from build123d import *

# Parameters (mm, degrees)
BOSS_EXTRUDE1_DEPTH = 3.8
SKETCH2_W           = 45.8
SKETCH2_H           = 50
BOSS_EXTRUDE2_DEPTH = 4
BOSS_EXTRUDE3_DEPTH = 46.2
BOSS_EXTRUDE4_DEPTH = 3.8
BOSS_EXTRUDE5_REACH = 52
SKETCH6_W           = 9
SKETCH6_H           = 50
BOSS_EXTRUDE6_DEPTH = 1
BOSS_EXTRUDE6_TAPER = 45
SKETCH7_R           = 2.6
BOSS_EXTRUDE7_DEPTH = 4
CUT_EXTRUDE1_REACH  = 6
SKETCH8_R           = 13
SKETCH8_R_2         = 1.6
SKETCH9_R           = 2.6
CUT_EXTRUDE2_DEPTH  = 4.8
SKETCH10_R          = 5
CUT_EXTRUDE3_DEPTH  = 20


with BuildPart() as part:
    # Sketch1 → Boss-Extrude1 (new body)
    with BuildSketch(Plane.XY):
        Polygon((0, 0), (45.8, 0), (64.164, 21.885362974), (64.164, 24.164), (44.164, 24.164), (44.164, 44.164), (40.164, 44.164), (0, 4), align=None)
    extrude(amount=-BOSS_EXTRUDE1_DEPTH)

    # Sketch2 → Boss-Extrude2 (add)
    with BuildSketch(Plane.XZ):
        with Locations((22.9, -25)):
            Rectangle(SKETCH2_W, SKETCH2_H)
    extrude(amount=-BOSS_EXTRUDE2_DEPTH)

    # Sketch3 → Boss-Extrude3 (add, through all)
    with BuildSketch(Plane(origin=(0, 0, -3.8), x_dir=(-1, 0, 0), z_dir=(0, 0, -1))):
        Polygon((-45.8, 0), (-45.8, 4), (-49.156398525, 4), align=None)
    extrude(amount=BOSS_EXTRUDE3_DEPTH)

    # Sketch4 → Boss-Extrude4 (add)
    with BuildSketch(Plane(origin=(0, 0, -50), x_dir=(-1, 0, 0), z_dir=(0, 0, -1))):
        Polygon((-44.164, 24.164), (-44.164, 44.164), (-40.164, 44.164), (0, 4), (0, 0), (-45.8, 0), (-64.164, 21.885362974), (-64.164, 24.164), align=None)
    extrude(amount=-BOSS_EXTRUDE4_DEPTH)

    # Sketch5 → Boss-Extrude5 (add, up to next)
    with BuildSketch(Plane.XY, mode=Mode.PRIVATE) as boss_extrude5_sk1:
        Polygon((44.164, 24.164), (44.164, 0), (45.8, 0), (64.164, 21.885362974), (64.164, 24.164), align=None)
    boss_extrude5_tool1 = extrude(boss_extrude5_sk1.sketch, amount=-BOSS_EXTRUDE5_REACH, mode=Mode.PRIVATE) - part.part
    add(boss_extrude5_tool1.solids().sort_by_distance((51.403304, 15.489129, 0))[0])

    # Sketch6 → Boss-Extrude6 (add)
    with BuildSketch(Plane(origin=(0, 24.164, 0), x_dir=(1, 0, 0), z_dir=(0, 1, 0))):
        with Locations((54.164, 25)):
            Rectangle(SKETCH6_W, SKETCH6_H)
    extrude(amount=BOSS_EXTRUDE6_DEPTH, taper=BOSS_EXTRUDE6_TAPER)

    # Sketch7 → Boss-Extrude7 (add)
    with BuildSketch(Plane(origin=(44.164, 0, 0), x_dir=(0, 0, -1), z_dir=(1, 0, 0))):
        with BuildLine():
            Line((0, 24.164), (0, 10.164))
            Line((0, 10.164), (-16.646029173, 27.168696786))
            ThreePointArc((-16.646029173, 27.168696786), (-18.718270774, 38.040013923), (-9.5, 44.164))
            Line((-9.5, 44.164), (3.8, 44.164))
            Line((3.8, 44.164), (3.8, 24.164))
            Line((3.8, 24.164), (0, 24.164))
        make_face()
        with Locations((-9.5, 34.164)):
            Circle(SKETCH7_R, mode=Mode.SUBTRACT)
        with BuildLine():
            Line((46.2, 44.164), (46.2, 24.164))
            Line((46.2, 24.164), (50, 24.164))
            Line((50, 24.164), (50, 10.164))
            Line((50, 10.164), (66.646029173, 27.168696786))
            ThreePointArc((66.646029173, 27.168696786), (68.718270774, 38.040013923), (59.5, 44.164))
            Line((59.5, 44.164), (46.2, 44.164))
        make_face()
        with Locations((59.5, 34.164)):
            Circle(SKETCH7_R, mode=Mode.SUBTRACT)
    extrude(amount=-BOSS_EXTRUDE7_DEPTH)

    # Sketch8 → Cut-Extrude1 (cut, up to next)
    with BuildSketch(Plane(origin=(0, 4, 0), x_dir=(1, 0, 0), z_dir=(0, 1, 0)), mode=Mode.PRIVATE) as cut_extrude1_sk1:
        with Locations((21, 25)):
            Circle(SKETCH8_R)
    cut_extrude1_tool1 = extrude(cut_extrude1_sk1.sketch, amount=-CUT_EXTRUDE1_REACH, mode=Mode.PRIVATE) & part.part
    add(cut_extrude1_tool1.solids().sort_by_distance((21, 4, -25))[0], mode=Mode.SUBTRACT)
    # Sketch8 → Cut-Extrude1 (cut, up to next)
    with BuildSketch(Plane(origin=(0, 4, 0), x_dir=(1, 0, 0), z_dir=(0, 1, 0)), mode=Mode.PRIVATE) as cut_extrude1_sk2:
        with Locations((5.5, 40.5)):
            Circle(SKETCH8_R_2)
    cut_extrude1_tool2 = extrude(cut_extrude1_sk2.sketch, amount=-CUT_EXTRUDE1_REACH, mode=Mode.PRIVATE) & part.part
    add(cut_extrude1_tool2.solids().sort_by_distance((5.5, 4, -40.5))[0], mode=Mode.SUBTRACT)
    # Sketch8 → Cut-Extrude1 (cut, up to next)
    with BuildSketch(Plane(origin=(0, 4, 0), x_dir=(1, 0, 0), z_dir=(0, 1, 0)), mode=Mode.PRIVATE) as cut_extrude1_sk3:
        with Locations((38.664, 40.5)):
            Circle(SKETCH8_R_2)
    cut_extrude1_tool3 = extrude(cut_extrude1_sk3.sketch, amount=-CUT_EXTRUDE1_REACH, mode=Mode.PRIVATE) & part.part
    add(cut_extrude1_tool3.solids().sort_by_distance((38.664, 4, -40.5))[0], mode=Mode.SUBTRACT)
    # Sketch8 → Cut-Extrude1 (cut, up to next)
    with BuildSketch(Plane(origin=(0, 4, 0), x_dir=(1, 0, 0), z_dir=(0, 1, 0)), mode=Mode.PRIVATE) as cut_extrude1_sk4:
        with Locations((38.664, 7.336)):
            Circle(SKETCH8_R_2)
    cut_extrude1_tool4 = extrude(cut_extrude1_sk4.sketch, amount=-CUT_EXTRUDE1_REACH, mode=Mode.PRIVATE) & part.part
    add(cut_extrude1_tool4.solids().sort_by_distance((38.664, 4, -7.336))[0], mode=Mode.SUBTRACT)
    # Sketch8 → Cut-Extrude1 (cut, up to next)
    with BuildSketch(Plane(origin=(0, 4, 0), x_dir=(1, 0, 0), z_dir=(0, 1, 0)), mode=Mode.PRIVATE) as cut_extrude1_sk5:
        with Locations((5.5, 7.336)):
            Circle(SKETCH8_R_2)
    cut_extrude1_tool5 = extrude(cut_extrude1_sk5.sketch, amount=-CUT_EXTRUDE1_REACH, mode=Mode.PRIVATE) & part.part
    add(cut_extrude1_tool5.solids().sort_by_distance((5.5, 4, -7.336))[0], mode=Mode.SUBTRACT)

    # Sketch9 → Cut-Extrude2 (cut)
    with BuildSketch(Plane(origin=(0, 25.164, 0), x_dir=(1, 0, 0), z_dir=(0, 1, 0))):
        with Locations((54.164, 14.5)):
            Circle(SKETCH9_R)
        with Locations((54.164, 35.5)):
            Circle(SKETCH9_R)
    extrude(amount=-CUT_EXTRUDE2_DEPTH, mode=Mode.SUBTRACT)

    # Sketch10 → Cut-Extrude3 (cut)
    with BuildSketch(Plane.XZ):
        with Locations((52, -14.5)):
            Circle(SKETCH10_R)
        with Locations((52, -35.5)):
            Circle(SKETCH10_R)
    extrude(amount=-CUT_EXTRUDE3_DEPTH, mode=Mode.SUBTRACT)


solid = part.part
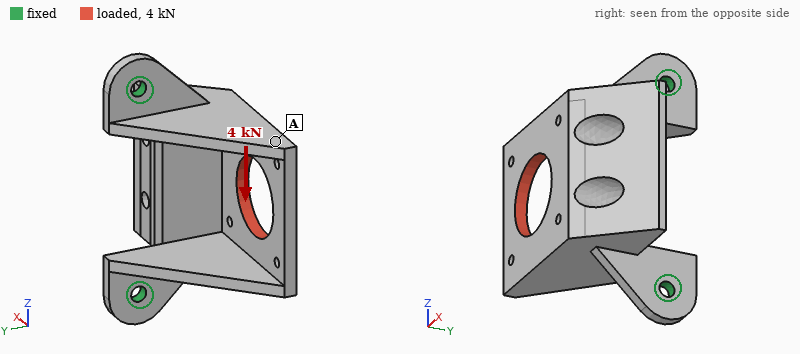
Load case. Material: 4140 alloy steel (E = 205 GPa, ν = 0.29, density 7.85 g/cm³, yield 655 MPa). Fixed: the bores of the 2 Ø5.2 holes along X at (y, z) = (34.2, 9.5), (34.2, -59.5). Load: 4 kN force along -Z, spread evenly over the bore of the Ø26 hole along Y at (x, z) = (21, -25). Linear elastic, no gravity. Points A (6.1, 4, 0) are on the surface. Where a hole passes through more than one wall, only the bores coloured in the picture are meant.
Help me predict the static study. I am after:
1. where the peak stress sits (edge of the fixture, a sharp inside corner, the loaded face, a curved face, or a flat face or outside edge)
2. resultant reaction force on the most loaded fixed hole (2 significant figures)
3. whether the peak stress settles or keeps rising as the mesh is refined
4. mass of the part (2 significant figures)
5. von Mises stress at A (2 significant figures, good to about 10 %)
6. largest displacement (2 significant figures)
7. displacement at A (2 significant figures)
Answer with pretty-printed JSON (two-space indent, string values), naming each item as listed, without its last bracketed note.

{
  "where the peak stress sits": "edge of the fixture",
  "resultant reaction force on the most loaded fixed hole": "2.8 kN",
  "whether the peak stress settles or keeps rising as the mesh is refined": "keeps rising",
  "mass of the part": "230 g",
  "von Mises stress at A": "70 MPa",
  "largest displacement": "0.20 mm",
  "displacement at A": "0.18 mm"
}
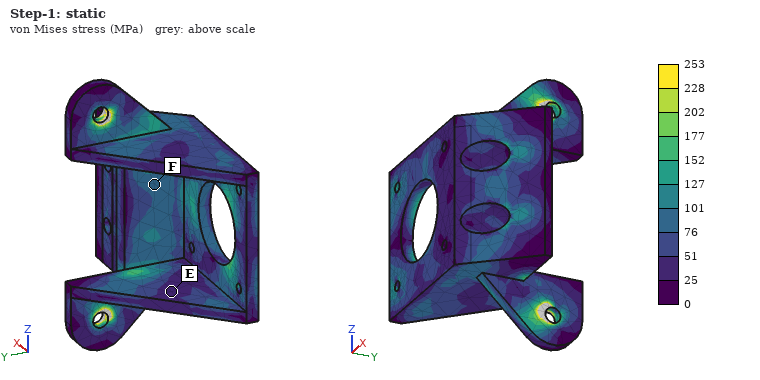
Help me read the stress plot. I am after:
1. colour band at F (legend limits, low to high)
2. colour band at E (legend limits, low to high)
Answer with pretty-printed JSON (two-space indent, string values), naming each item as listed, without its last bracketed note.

{
  "colour band at F": "76 to 101 MPa",
  "colour band at E": "25 to 51 MPa"
}
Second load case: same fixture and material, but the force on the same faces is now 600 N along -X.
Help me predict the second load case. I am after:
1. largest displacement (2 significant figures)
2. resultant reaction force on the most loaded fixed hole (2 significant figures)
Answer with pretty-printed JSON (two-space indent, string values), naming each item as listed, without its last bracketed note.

{
  "largest displacement": "0.11 mm",
  "resultant reaction force on the most loaded fixed hole": "310 N"
}
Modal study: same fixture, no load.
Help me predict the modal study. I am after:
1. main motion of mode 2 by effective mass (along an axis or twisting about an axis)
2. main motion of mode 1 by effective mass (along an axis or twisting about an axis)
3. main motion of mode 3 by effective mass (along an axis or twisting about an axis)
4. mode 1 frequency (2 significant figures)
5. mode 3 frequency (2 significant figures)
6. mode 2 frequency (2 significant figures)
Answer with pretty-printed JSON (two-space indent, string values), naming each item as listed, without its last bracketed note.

{
  "main motion of mode 2 by effective mass": "along Z",
  "main motion of mode 1 by effective mass": "along X",
  "main motion of mode 3 by effective mass": "along X",
  "mode 1 frequency": "1200 Hz",
  "mode 3 frequency": "5500 Hz",
  "mode 2 frequency": "2700 Hz"
}
